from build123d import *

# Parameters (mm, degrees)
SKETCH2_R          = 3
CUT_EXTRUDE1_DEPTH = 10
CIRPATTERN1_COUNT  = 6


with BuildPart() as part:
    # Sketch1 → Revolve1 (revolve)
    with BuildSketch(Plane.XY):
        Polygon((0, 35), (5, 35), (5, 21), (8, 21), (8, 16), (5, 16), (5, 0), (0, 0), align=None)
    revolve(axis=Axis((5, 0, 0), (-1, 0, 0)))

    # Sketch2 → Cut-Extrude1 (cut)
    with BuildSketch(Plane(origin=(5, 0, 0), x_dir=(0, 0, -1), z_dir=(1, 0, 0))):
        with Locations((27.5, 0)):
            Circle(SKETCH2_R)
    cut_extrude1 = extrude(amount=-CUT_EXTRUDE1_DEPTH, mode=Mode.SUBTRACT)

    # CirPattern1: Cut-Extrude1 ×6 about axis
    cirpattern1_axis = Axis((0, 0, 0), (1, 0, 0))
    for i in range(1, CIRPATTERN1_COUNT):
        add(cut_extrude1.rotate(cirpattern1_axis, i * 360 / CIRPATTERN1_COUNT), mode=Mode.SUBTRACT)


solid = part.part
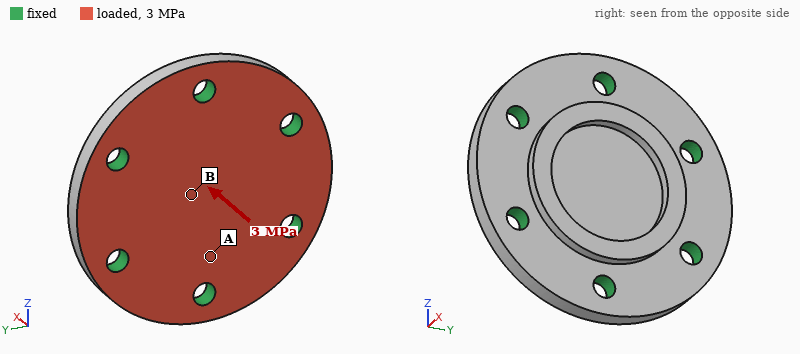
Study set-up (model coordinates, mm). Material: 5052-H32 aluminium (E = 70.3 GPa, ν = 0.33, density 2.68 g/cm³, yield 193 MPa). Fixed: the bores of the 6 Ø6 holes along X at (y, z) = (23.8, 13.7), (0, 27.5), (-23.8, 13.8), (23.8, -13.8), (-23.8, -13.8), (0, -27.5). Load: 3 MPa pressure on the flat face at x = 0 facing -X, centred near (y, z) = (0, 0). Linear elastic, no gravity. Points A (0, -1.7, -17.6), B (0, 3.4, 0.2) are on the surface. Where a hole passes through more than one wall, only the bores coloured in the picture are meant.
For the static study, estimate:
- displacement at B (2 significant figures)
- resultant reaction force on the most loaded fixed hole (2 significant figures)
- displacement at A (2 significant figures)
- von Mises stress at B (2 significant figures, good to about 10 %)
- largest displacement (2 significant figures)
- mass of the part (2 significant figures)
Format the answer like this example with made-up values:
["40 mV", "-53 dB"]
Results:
["29 µm", "1.8 kN", "12 µm", "34 MPa", "30 µm", "54 g"]
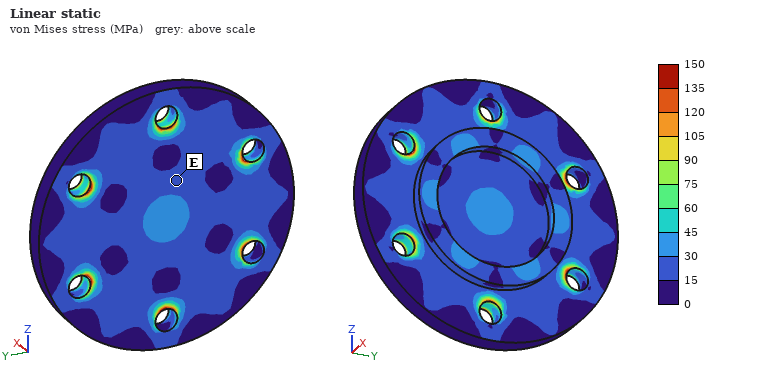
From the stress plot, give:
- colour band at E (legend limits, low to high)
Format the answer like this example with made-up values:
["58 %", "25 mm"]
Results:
["15 to 30 MPa"]
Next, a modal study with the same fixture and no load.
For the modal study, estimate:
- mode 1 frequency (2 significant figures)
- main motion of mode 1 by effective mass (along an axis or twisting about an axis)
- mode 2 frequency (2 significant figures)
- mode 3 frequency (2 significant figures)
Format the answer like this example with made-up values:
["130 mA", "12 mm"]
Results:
["16 kHz", "along X", "28 kHz", "28 kHz"]
